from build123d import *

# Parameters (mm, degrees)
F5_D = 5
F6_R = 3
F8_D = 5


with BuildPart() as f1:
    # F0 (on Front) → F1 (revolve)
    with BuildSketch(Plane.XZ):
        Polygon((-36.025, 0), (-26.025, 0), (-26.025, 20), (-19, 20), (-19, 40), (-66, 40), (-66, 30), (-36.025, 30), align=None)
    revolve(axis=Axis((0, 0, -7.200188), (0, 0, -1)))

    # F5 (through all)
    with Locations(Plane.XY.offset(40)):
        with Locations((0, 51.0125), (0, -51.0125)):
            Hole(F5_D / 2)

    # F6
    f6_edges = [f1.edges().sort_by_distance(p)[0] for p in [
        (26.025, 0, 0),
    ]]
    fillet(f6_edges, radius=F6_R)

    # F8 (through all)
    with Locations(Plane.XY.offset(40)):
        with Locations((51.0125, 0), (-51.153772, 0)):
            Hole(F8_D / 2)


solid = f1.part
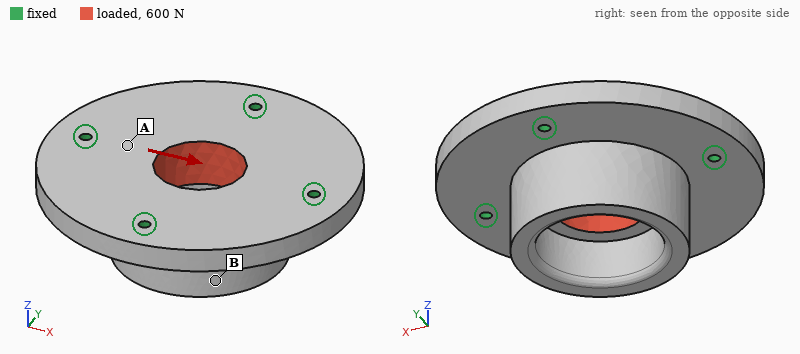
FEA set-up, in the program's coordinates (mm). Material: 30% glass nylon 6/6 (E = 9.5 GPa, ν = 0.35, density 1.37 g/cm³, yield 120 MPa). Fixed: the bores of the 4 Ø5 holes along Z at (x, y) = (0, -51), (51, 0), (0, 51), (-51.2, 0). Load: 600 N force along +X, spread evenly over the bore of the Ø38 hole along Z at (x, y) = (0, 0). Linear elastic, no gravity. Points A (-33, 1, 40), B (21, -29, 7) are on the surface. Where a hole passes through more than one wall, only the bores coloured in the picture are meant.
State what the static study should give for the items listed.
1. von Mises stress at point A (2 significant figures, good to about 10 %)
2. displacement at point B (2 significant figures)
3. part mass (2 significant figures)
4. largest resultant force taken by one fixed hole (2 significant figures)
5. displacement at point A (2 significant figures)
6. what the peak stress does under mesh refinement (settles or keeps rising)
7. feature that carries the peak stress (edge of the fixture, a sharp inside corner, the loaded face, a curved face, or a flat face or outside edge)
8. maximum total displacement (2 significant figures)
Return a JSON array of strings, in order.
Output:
["0.41 MPa", "2.7 µm", "260 g", "180 N", "1.6 µm", "keeps rising", "edge of the fixture", "2.9 µm"]
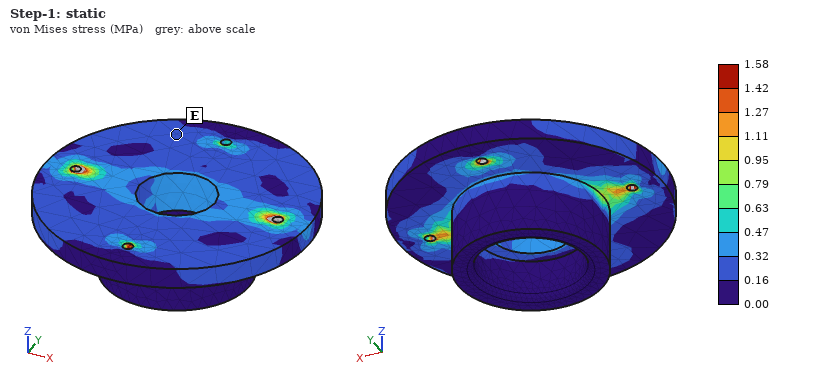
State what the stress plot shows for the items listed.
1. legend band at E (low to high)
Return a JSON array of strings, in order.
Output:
["0.16 to 0.32 MPa"]
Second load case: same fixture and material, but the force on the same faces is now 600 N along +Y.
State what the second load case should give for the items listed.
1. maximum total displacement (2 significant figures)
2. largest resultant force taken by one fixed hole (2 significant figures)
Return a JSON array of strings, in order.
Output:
["2.9 µm", "180 N"]
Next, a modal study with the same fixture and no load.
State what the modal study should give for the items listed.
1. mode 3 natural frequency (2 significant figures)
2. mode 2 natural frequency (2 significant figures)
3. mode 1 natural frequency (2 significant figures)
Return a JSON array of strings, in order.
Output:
["3200 Hz", "3200 Hz", "3200 Hz"]
